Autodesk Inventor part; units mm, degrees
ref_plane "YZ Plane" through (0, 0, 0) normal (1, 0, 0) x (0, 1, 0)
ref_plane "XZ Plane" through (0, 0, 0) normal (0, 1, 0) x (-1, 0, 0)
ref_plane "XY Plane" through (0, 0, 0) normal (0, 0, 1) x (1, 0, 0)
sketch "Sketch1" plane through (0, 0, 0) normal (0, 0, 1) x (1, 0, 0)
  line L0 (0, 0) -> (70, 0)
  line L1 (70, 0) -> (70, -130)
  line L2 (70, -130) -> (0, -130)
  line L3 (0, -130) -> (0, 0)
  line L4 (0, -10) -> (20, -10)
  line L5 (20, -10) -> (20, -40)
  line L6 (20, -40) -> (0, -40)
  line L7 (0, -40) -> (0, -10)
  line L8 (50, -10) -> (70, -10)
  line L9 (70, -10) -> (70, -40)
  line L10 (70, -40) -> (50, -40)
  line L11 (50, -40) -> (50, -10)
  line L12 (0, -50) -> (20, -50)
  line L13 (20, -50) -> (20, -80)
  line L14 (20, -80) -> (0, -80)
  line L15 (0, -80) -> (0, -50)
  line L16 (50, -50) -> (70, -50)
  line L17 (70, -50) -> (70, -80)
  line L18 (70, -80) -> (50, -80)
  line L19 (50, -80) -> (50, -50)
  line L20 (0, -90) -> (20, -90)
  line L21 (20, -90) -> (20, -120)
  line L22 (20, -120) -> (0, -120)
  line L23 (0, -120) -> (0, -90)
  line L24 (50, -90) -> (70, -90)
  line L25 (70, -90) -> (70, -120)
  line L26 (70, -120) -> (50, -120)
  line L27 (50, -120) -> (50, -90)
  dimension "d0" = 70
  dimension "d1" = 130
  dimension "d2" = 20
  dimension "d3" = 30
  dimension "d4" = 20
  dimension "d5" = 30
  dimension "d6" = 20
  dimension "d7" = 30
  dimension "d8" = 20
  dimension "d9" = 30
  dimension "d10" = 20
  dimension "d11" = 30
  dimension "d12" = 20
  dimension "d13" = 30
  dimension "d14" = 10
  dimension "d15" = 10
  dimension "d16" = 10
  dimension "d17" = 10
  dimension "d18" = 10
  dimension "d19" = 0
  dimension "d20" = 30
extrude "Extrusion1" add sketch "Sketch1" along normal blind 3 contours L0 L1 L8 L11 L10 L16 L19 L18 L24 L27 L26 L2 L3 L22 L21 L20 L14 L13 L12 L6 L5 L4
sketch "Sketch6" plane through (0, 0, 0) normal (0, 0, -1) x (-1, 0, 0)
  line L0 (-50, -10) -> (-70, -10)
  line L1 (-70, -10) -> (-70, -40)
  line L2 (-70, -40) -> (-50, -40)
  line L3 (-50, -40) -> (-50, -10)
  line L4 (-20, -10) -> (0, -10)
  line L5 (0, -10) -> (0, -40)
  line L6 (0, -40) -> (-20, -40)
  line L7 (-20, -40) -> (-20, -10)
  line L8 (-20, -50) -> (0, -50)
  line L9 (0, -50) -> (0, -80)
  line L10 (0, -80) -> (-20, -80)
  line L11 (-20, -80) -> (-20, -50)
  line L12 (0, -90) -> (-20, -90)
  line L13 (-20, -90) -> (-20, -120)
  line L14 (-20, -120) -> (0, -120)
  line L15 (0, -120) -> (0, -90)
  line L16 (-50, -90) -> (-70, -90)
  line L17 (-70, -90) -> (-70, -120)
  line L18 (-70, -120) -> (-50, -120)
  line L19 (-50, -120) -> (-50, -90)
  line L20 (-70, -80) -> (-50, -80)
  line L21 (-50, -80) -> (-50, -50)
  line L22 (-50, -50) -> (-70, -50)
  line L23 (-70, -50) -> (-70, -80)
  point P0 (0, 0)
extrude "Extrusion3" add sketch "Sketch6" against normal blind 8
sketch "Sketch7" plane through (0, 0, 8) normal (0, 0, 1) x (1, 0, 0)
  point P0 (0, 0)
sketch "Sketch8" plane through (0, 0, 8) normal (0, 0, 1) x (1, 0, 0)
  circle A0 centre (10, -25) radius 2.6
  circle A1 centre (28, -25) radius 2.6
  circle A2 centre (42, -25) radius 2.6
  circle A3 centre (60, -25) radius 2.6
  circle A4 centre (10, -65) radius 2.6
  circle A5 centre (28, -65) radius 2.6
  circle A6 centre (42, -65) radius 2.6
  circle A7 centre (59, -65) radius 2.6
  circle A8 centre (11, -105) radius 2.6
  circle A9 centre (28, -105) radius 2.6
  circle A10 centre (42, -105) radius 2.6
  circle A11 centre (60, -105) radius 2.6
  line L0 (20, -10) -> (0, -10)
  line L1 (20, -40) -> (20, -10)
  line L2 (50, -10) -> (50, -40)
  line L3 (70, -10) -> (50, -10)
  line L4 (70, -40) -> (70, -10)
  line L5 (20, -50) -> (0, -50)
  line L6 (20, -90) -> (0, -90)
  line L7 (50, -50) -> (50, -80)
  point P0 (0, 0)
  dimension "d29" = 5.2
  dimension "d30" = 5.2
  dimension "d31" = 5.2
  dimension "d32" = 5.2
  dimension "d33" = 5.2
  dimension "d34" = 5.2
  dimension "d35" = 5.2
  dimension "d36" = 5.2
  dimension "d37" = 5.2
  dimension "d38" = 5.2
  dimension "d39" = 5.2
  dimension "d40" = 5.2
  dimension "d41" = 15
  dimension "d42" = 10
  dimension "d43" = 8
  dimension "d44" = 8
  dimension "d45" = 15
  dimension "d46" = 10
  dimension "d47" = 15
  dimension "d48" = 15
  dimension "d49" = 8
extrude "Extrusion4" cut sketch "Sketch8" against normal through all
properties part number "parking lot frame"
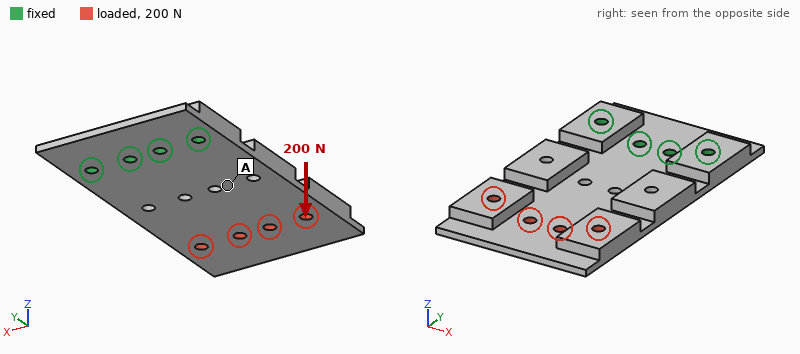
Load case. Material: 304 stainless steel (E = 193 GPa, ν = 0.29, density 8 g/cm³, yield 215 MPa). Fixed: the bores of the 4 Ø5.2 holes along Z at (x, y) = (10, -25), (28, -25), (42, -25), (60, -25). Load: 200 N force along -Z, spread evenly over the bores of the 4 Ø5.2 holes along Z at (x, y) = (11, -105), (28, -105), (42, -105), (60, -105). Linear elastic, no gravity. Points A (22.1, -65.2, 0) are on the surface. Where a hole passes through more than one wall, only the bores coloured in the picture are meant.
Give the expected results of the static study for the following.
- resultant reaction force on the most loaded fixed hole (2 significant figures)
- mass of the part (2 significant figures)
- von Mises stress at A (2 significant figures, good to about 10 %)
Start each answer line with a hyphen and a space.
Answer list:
- 400 N
- 350 g
- 19 MPa
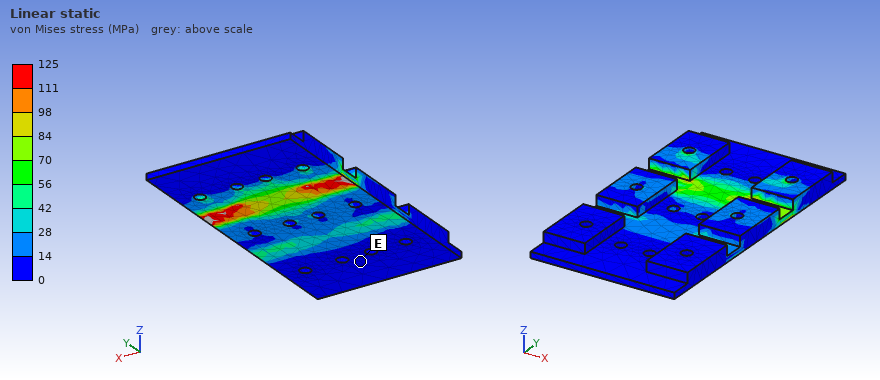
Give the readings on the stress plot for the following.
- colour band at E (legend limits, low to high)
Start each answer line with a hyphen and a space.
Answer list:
- 0 to 14 MPa
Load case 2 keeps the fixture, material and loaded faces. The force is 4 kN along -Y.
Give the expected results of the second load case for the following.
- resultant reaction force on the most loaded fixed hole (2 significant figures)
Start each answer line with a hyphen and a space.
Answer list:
- 1.5 kN
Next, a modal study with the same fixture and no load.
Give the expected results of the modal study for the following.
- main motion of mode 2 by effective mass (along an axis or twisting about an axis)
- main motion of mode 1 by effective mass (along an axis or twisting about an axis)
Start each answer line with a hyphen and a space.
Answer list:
- twisting about Y
- along Z
